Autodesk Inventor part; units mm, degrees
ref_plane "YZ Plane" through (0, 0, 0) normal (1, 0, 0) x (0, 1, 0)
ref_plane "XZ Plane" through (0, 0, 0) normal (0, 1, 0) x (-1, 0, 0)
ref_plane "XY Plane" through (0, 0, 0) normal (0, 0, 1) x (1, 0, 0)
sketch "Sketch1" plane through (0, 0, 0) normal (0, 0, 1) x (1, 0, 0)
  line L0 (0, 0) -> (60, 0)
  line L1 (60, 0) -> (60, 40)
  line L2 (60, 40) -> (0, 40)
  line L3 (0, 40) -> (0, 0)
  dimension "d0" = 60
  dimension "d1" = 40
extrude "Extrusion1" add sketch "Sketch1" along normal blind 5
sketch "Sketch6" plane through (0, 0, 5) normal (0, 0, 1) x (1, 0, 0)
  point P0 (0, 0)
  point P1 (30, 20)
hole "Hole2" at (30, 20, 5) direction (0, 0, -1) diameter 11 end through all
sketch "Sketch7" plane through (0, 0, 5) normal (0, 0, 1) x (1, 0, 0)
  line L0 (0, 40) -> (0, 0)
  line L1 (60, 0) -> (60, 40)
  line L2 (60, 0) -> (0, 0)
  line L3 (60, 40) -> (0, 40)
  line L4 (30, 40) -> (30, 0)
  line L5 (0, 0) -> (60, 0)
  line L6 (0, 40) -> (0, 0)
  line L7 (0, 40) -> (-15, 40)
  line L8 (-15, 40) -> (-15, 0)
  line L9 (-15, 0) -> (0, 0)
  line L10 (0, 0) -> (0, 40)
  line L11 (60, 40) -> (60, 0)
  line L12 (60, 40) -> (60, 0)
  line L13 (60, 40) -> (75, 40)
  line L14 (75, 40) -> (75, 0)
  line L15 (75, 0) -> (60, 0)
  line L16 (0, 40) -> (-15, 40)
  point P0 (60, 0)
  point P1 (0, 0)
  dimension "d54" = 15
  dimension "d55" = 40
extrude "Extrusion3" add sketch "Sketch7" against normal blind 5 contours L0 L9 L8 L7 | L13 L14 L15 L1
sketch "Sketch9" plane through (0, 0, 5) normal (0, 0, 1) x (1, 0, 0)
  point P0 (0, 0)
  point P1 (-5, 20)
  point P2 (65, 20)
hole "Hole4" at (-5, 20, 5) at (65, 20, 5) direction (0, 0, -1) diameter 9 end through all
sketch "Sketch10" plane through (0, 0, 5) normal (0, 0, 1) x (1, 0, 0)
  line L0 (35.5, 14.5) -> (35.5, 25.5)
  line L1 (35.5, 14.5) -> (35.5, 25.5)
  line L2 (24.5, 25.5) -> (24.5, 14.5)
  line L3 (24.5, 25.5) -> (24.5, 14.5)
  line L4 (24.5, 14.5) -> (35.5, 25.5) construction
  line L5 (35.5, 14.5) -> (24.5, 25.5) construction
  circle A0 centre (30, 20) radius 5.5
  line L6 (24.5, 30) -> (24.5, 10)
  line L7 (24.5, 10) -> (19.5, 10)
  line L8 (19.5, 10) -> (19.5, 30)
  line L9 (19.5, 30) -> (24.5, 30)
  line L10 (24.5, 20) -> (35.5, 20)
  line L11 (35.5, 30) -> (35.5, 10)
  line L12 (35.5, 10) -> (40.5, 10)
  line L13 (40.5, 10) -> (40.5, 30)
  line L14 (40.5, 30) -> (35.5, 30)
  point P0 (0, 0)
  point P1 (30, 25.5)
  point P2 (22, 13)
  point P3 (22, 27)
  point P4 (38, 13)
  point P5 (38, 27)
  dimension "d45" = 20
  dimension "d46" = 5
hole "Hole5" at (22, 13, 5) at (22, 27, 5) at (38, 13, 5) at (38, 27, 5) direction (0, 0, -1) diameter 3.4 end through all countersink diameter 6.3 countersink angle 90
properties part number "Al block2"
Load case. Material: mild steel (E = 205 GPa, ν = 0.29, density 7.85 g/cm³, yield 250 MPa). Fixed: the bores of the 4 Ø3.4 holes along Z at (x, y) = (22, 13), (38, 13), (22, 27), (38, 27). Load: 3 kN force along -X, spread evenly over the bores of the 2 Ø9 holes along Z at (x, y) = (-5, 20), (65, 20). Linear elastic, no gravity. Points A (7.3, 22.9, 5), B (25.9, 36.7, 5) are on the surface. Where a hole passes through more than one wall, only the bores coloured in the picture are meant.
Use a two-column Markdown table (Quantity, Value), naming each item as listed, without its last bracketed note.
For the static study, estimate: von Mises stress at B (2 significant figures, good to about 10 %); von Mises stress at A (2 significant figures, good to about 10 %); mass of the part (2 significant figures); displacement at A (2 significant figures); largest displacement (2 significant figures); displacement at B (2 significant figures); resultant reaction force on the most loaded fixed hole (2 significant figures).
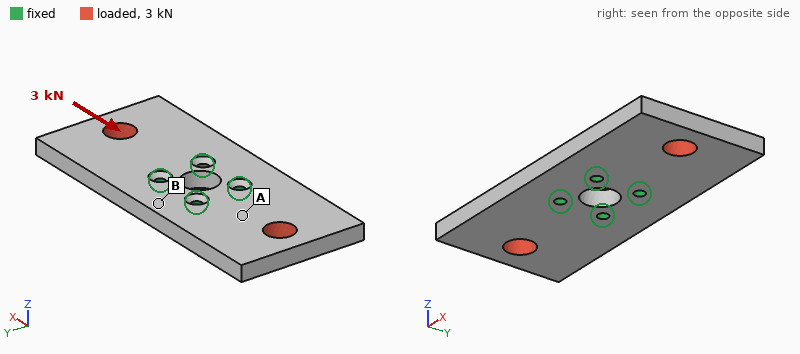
| Quantity | Value |
|---|---|
| von Mises stress at B | 3.7 MPa |
| von Mises stress at A | 12 MPa |
| mass of the part | 130 g |
| displacement at A | 1.2 µm |
| largest displacement | 2.9 µm |
| displacement at B | 0.52 µm |
| resultant reaction force on the most loaded fixed hole | 770 N |
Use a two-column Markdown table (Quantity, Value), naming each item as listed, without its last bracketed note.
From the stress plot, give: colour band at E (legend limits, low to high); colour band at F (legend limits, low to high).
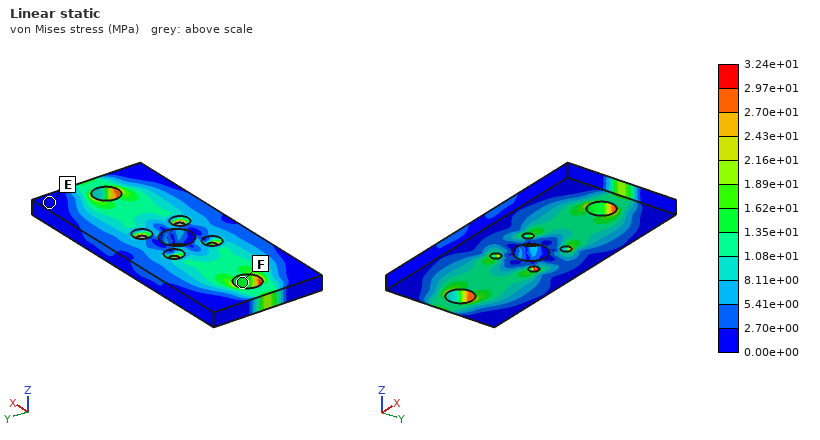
| Quantity | Value |
|---|---|
| colour band at E | 0.00e+00 to 2.70e+00 MPa |
| colour band at F | 1.35e+01 to 1.62e+01 MPa |
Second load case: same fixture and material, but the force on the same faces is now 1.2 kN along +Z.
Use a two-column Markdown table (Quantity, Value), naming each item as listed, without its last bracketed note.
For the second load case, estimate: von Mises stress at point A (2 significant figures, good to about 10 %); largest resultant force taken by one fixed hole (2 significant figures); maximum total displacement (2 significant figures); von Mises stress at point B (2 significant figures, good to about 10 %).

| Quantity | Value |
|---|---|
| von Mises stress at point A | 44 MPa |
| largest resultant force taken by one fixed hole | 440 N |
| maximum total displacement | 94 µm |
| von Mises stress at point B | 48 MPa |
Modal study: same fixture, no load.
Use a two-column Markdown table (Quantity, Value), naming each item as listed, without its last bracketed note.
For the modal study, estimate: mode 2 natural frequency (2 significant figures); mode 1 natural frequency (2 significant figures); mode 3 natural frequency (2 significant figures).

| Quantity | Value |
|---|---|
| mode 2 natural frequency | 2800 Hz |
| mode 1 natural frequency | 2800 Hz |
| mode 3 natural frequency | 5500 Hz |
